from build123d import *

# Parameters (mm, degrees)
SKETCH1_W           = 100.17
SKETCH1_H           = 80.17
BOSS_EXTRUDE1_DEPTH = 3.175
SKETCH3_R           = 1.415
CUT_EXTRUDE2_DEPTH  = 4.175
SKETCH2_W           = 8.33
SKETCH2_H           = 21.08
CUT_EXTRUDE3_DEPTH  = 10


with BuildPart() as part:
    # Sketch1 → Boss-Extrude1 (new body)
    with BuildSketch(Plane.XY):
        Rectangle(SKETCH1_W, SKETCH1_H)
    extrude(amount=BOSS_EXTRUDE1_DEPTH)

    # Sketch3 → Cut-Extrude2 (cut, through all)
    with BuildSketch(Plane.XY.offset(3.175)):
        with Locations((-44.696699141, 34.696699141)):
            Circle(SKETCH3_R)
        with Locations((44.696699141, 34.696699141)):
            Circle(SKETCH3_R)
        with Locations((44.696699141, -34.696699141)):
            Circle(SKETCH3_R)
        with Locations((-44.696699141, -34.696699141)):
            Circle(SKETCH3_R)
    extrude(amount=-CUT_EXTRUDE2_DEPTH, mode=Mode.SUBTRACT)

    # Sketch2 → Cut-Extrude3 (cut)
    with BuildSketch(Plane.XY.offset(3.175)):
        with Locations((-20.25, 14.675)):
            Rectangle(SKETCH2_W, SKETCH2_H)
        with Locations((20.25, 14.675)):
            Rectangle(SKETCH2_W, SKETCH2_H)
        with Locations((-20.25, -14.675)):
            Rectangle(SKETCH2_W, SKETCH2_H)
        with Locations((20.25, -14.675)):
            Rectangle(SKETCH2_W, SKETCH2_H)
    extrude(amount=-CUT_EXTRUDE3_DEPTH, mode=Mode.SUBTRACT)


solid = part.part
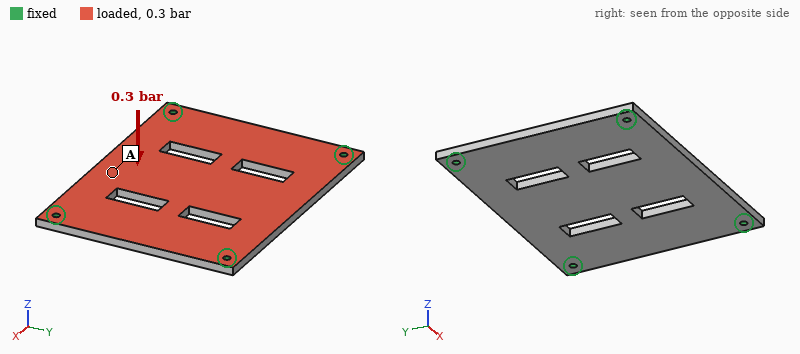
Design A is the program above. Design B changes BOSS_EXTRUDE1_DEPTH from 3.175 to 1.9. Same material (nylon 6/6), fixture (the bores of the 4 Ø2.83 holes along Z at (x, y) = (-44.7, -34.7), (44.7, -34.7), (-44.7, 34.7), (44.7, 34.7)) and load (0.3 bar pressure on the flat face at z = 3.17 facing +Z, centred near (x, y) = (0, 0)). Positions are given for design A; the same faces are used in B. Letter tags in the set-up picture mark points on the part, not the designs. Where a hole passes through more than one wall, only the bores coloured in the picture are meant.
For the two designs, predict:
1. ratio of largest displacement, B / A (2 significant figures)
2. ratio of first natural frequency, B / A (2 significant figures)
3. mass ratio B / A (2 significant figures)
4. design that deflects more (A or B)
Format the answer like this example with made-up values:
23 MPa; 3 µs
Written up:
4.4; 0.62; 0.60; B
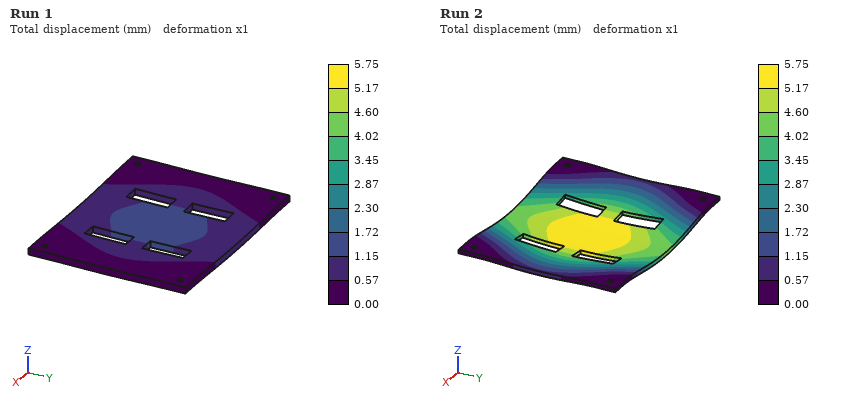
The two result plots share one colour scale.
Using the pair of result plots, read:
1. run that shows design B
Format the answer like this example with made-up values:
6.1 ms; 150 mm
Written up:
Run 2
